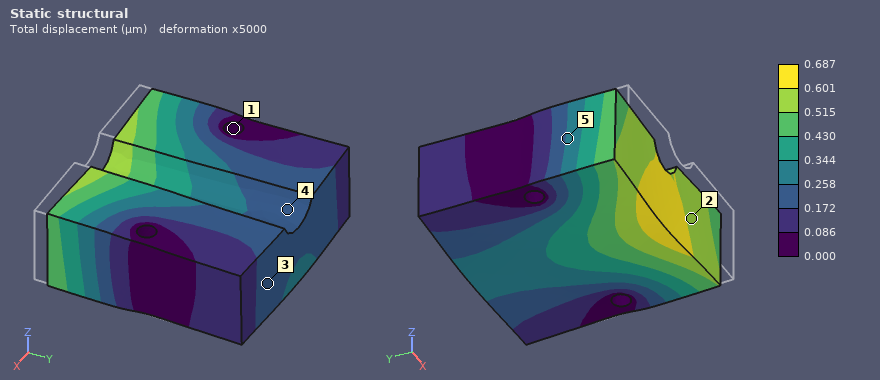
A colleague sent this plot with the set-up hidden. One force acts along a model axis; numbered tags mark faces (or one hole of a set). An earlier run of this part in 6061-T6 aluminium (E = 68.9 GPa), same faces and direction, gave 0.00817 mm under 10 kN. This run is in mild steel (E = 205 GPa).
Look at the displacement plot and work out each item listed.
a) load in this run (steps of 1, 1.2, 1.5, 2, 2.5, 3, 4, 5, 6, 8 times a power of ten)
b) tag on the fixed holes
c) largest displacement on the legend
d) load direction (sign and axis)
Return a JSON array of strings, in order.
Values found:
["2.5 kN", "1", "0.687 µm", "+Y"]
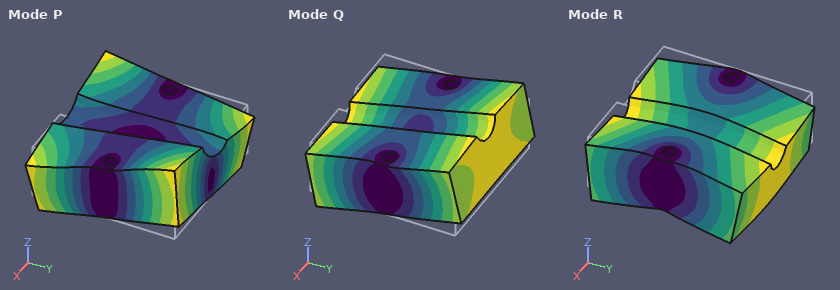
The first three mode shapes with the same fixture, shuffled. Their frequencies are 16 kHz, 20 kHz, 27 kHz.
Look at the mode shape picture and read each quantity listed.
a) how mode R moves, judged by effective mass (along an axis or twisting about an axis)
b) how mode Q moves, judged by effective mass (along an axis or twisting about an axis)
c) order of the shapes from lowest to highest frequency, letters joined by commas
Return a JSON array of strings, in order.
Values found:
["along Z", "twisting about X", "Q, R, P"]
